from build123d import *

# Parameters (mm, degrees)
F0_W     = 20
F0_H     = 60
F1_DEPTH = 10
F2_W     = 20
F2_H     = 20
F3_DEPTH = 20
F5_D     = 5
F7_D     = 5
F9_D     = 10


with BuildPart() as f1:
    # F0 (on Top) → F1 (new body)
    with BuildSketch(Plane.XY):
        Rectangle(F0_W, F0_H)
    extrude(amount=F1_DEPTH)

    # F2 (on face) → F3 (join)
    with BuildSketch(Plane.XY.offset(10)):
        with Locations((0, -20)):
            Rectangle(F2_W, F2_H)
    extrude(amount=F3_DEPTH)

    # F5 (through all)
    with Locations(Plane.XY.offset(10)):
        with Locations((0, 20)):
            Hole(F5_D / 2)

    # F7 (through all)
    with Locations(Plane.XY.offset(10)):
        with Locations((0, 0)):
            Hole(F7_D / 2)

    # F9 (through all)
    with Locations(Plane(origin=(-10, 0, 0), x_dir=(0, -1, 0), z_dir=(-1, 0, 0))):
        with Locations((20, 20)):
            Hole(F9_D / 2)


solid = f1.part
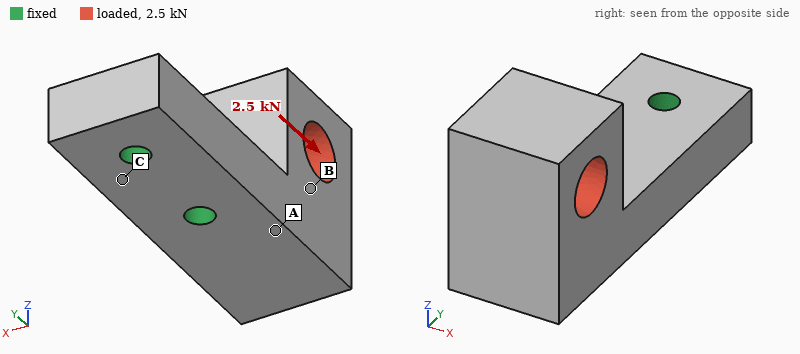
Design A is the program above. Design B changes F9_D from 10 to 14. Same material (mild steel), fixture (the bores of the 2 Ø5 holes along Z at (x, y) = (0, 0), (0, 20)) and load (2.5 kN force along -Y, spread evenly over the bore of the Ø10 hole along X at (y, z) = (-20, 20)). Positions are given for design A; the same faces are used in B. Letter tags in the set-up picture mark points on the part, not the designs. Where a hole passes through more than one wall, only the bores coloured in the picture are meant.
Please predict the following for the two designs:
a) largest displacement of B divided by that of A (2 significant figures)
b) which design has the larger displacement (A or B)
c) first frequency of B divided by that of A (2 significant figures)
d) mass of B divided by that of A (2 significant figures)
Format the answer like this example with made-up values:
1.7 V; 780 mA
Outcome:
1.1; B; 1.1; 0.92
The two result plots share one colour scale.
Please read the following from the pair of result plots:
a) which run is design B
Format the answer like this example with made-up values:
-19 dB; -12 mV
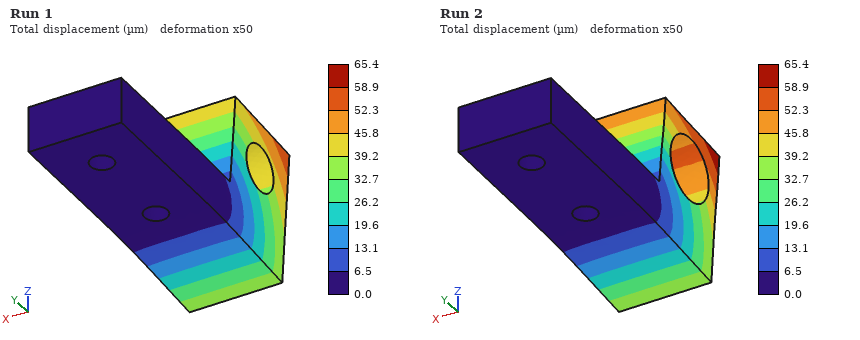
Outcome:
Run 2
